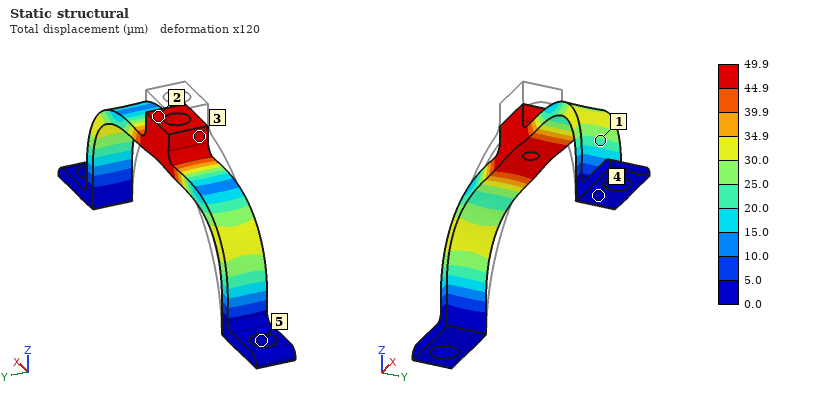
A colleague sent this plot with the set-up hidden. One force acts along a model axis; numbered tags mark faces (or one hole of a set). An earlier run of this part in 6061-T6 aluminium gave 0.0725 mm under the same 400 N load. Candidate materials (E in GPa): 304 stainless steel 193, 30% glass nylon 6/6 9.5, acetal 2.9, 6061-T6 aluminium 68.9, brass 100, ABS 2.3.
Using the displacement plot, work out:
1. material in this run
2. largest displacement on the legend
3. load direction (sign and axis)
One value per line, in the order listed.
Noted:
brass
49.9 µm
-Z
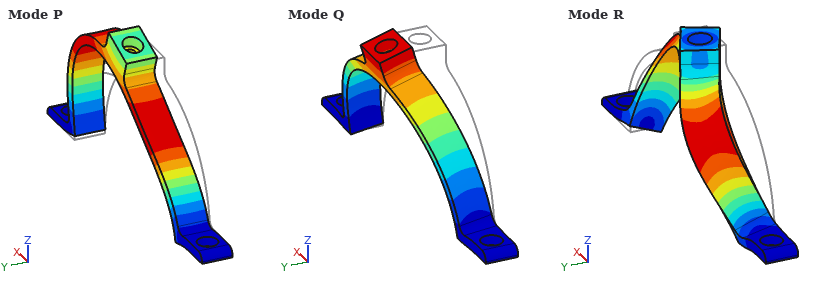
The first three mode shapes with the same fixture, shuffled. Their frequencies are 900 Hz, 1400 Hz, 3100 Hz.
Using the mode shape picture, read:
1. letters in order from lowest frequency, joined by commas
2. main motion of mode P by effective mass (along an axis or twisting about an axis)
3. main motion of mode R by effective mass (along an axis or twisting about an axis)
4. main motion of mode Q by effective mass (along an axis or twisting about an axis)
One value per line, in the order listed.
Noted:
Q, P, R
along X
twisting about Z
along Y
